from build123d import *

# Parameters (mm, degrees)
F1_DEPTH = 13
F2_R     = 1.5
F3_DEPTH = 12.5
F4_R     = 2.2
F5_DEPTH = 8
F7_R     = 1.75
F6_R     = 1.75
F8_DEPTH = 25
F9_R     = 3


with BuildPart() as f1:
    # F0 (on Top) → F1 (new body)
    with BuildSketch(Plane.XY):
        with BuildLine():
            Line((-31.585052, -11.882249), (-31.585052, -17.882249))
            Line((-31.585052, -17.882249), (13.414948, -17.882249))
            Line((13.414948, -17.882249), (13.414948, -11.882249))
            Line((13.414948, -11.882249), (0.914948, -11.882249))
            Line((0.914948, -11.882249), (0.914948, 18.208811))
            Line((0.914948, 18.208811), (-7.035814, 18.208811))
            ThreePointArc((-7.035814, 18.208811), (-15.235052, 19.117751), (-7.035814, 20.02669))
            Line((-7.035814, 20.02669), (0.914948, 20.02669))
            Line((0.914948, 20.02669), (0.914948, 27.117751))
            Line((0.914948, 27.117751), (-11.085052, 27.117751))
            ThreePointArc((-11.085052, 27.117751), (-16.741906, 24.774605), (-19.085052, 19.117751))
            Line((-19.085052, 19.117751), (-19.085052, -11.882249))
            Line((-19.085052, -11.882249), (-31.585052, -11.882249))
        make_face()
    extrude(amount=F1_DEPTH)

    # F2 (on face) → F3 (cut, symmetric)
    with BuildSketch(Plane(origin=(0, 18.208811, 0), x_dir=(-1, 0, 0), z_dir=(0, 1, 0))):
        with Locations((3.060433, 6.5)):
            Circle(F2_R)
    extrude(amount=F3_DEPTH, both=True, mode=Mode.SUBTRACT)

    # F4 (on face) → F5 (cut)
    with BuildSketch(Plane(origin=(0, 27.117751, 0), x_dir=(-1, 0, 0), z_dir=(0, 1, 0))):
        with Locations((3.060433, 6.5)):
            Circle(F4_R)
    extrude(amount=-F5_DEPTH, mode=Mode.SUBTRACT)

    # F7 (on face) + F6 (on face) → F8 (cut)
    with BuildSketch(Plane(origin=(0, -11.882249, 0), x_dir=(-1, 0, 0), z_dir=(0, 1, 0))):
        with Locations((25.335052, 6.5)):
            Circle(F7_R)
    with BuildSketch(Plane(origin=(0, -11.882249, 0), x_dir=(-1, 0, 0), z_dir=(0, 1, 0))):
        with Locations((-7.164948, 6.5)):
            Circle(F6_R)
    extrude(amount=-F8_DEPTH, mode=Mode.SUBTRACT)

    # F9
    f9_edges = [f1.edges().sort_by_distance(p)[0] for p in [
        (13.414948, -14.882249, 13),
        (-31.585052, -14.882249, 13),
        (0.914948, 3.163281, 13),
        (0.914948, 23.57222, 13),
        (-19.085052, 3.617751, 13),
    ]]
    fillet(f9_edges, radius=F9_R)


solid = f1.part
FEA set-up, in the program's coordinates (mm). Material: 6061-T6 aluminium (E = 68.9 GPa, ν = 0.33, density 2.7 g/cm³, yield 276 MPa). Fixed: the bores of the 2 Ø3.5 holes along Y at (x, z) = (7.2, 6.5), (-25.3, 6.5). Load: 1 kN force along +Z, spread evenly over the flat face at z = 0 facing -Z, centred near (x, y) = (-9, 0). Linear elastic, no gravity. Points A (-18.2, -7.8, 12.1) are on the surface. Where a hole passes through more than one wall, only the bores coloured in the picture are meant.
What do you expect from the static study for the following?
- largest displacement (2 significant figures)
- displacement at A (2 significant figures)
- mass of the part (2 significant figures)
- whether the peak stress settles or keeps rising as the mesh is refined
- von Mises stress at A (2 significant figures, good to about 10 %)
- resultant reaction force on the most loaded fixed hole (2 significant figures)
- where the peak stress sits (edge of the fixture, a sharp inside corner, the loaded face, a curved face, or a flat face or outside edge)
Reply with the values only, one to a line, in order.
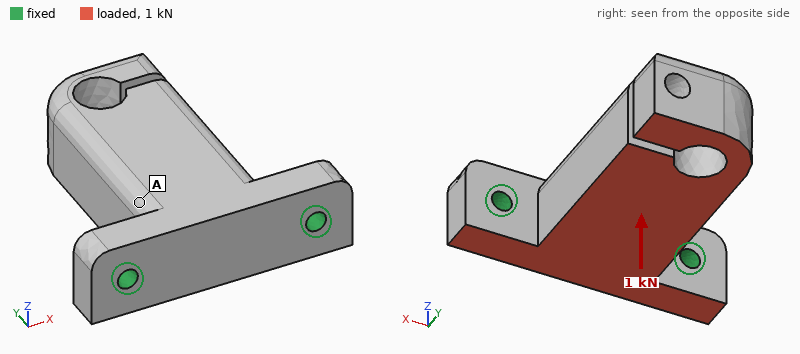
0.19 mm
0.033 mm
33 g
keeps rising
23 MPa
500 N
edge of the fixture
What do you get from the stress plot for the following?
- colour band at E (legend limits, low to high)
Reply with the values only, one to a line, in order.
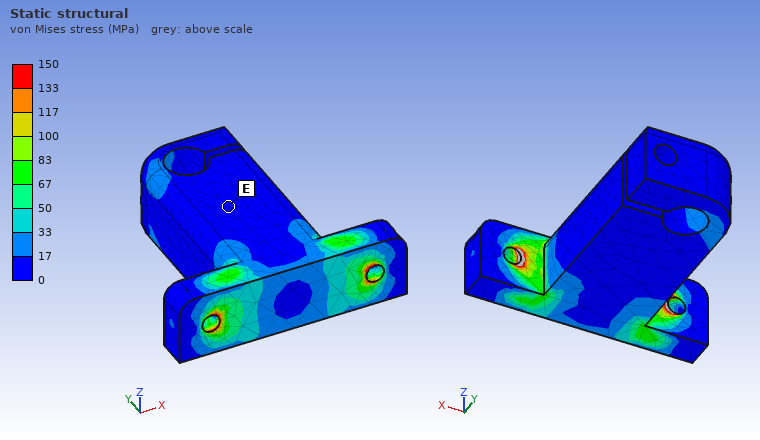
0 to 17 MPa
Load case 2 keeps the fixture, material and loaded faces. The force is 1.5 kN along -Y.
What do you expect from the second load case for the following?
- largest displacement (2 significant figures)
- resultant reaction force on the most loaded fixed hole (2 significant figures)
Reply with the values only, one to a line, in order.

0.15 mm
790 N
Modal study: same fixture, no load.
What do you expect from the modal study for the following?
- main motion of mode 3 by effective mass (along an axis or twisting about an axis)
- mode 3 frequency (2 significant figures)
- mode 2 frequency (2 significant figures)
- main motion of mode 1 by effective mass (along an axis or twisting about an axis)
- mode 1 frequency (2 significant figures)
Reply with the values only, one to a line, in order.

along X
6800 Hz
4500 Hz
along Z
2700 Hz
